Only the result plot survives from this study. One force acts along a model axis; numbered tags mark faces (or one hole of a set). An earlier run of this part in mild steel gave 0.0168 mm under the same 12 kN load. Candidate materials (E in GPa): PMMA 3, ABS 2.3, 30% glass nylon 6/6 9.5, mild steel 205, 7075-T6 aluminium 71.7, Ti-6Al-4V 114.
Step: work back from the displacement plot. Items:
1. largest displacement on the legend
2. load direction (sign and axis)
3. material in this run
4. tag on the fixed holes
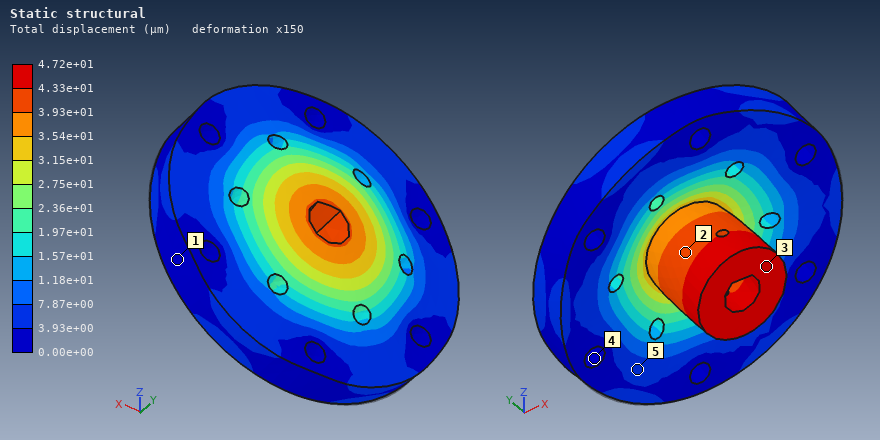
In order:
4.72e+01 µm
+Y
7075-T6 aluminium
4
